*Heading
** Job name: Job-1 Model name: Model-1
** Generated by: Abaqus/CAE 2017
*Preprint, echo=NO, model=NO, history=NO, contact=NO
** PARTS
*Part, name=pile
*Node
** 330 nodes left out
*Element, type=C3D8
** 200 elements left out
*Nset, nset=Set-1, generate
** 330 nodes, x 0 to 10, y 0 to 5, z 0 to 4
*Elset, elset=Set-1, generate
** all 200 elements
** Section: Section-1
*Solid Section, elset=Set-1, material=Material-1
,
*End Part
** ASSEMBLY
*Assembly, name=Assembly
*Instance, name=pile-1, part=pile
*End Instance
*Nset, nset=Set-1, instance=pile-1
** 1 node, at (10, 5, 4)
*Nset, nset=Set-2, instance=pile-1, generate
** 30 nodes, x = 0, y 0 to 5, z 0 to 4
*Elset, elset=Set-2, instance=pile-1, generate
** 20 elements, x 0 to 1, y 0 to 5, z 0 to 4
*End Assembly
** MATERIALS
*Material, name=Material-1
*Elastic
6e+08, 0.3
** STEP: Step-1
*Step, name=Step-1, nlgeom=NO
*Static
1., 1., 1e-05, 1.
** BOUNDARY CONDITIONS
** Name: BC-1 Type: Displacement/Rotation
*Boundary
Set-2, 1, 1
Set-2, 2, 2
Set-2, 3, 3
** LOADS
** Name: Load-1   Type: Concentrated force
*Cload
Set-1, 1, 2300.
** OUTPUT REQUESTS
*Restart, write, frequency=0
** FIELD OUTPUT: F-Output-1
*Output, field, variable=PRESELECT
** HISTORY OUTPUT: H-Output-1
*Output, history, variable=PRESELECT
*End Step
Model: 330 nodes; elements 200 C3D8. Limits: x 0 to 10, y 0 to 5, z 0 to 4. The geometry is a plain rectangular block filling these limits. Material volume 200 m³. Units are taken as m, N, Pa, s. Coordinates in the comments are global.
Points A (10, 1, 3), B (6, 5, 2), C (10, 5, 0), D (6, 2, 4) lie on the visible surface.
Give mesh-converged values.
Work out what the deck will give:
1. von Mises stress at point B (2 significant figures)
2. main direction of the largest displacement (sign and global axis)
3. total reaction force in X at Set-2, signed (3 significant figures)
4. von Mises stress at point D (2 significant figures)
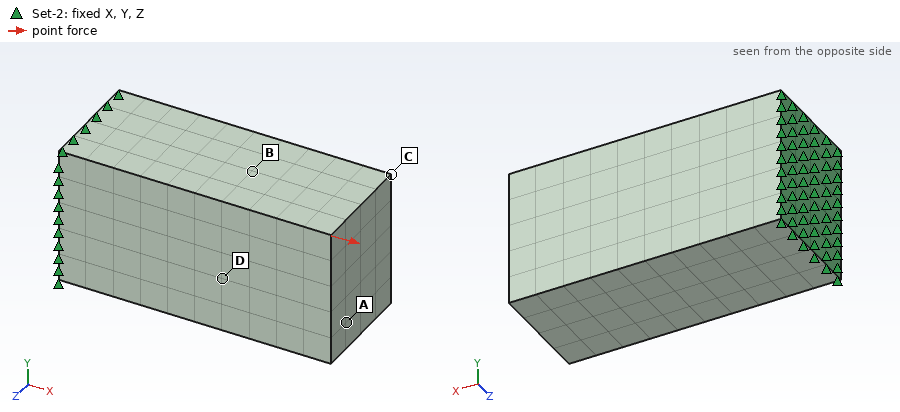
450 Pa
+X
-2300 N
320 Pa
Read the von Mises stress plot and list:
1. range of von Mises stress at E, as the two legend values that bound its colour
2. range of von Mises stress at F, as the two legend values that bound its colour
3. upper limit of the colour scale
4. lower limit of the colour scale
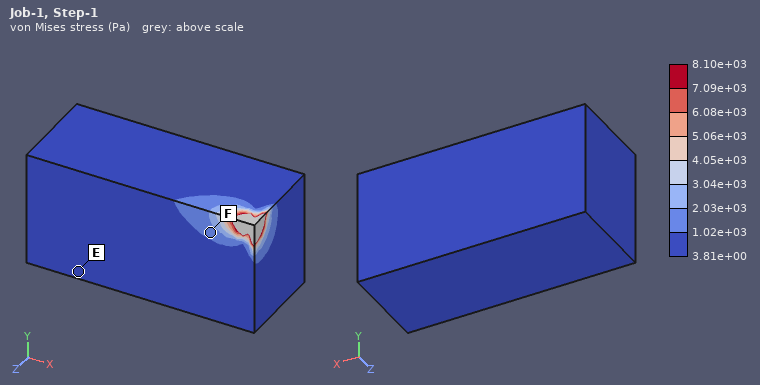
3.81e+00 to 1.02e+03 Pa
1.02e+03 to 2.03e+03 Pa
8.10e+03 Pa
3.81e+00 Pa
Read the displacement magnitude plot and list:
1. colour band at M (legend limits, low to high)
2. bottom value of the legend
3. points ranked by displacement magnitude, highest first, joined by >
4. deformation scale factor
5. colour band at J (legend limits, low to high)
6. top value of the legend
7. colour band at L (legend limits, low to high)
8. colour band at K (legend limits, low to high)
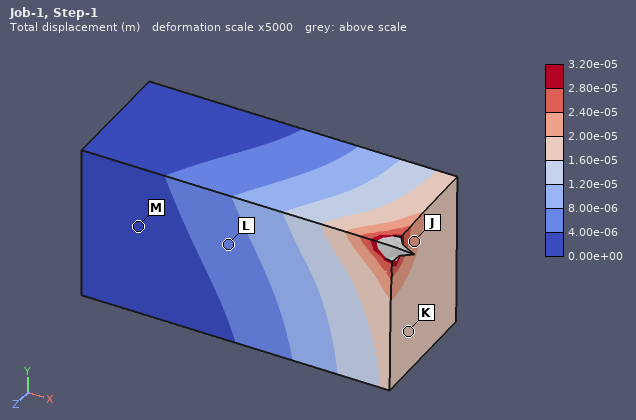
0.00e+00 to 4.00e-06 m
0.00e+00 m
J > K > L > M
5000
2.00e-05 to 2.40e-05 m
3.20e-05 m
4.00e-06 to 8.00e-06 m
1.60e-05 to 2.00e-05 m
